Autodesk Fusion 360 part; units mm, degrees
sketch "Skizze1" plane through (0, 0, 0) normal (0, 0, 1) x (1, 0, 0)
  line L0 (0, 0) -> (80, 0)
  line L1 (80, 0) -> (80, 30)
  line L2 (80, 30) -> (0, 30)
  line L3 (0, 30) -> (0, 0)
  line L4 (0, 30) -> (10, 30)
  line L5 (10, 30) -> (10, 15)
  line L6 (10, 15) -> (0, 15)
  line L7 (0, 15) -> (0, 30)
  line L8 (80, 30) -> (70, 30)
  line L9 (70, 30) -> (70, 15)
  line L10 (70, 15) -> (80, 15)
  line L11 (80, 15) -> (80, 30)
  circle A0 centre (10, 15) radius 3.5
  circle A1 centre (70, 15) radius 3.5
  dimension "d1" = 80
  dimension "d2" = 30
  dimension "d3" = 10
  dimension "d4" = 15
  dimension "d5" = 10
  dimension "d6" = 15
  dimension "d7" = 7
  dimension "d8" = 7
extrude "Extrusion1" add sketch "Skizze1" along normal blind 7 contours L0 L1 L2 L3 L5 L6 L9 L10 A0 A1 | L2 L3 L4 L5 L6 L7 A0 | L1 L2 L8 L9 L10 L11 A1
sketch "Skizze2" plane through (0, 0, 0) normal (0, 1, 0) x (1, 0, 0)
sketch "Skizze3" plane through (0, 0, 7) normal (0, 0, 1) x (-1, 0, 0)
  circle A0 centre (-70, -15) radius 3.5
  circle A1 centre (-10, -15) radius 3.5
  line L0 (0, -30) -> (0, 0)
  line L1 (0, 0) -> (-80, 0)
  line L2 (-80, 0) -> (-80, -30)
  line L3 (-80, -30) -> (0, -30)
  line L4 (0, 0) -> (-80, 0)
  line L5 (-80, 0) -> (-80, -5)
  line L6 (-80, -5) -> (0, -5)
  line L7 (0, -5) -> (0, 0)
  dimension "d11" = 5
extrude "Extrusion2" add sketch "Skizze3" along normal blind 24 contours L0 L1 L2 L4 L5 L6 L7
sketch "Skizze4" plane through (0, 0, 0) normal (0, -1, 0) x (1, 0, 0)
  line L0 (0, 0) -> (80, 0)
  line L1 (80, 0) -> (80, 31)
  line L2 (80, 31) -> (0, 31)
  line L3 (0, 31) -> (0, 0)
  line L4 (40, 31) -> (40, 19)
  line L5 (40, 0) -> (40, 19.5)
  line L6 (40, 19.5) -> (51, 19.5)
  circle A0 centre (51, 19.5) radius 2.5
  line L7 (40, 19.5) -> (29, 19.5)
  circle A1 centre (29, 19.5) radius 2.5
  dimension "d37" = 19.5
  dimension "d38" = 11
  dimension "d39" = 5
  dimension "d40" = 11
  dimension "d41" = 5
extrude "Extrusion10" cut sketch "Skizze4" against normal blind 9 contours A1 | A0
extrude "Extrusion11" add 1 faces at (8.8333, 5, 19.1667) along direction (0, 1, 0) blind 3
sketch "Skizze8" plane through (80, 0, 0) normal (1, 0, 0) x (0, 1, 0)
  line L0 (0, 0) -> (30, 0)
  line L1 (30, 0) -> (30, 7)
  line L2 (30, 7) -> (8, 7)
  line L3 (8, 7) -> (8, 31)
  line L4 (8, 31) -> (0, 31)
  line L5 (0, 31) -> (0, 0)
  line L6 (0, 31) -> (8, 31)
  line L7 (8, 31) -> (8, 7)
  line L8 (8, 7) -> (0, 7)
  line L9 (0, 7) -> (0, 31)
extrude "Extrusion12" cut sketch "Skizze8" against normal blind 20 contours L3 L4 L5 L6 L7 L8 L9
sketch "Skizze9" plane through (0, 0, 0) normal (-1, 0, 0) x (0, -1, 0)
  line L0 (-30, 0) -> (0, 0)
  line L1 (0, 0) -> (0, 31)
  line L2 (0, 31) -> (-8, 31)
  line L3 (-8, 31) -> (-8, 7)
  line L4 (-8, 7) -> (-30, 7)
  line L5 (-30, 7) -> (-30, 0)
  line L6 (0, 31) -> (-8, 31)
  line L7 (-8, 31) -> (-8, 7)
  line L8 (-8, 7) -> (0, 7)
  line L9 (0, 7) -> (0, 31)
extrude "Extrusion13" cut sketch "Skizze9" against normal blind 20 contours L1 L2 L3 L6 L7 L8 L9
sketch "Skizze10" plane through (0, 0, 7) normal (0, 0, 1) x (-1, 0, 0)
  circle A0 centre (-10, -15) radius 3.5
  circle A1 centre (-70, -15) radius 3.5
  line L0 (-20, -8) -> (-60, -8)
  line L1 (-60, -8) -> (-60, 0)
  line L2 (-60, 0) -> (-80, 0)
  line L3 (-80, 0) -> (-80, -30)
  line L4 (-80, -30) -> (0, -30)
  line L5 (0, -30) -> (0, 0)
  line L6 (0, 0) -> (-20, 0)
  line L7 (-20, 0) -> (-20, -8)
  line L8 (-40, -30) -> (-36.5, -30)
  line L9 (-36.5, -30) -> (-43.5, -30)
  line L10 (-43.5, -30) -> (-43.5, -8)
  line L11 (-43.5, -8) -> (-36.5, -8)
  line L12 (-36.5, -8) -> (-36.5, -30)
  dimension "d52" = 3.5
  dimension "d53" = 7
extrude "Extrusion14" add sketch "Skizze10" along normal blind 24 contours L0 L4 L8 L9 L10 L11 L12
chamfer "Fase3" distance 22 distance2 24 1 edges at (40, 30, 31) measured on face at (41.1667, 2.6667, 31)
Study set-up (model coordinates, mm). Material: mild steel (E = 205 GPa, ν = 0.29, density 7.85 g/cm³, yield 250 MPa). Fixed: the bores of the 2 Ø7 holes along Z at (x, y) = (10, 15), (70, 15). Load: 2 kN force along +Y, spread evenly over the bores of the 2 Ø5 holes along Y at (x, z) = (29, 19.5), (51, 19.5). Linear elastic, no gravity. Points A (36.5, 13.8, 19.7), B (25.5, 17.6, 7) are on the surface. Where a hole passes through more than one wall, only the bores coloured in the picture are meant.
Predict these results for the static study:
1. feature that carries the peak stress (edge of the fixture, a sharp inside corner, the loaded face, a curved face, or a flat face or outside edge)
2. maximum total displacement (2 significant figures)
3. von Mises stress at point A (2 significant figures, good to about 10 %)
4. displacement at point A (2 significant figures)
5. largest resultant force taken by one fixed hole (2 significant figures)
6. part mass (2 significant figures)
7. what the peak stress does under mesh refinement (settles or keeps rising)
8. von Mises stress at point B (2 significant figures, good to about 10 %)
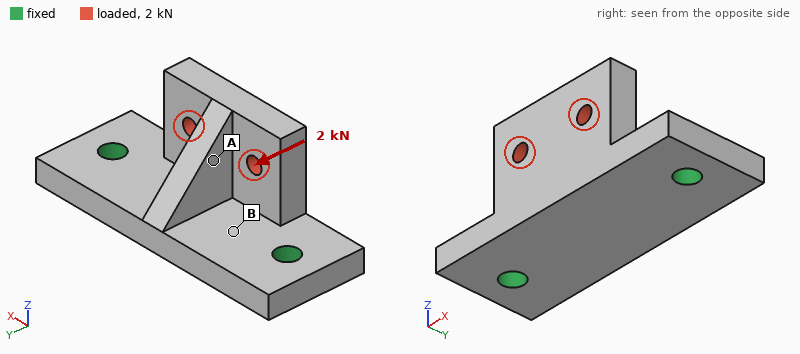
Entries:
edge of the fixture
38 µm
14 MPa
21 µm
1.0 kN
200 g
keeps rising
40 MPa
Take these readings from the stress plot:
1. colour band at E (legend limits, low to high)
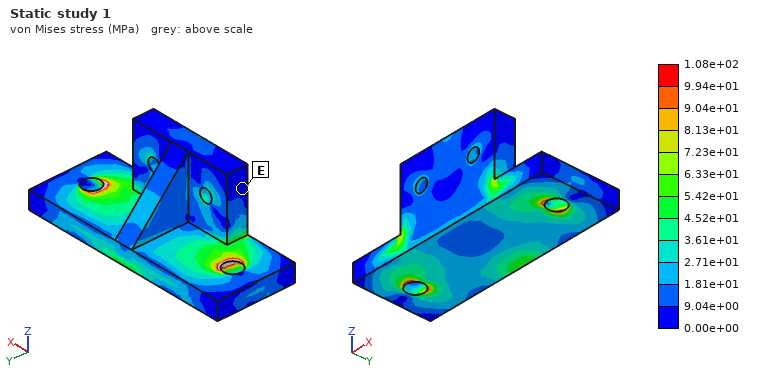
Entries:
0.00e+00 to 9.04e+00 MPa
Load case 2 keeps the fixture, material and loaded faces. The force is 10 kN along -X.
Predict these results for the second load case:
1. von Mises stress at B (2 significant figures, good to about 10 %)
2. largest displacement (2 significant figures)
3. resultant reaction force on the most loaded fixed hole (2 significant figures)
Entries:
59 MPa
36 µm
6.3 kN
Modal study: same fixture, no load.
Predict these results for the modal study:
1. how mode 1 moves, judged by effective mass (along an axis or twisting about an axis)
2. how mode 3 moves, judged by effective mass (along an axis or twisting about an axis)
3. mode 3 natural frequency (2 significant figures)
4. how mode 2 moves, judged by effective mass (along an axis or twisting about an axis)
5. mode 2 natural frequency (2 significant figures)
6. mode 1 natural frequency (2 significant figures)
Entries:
along Y
along X
11 kHz
along Z
8600 Hz
4900 Hz
